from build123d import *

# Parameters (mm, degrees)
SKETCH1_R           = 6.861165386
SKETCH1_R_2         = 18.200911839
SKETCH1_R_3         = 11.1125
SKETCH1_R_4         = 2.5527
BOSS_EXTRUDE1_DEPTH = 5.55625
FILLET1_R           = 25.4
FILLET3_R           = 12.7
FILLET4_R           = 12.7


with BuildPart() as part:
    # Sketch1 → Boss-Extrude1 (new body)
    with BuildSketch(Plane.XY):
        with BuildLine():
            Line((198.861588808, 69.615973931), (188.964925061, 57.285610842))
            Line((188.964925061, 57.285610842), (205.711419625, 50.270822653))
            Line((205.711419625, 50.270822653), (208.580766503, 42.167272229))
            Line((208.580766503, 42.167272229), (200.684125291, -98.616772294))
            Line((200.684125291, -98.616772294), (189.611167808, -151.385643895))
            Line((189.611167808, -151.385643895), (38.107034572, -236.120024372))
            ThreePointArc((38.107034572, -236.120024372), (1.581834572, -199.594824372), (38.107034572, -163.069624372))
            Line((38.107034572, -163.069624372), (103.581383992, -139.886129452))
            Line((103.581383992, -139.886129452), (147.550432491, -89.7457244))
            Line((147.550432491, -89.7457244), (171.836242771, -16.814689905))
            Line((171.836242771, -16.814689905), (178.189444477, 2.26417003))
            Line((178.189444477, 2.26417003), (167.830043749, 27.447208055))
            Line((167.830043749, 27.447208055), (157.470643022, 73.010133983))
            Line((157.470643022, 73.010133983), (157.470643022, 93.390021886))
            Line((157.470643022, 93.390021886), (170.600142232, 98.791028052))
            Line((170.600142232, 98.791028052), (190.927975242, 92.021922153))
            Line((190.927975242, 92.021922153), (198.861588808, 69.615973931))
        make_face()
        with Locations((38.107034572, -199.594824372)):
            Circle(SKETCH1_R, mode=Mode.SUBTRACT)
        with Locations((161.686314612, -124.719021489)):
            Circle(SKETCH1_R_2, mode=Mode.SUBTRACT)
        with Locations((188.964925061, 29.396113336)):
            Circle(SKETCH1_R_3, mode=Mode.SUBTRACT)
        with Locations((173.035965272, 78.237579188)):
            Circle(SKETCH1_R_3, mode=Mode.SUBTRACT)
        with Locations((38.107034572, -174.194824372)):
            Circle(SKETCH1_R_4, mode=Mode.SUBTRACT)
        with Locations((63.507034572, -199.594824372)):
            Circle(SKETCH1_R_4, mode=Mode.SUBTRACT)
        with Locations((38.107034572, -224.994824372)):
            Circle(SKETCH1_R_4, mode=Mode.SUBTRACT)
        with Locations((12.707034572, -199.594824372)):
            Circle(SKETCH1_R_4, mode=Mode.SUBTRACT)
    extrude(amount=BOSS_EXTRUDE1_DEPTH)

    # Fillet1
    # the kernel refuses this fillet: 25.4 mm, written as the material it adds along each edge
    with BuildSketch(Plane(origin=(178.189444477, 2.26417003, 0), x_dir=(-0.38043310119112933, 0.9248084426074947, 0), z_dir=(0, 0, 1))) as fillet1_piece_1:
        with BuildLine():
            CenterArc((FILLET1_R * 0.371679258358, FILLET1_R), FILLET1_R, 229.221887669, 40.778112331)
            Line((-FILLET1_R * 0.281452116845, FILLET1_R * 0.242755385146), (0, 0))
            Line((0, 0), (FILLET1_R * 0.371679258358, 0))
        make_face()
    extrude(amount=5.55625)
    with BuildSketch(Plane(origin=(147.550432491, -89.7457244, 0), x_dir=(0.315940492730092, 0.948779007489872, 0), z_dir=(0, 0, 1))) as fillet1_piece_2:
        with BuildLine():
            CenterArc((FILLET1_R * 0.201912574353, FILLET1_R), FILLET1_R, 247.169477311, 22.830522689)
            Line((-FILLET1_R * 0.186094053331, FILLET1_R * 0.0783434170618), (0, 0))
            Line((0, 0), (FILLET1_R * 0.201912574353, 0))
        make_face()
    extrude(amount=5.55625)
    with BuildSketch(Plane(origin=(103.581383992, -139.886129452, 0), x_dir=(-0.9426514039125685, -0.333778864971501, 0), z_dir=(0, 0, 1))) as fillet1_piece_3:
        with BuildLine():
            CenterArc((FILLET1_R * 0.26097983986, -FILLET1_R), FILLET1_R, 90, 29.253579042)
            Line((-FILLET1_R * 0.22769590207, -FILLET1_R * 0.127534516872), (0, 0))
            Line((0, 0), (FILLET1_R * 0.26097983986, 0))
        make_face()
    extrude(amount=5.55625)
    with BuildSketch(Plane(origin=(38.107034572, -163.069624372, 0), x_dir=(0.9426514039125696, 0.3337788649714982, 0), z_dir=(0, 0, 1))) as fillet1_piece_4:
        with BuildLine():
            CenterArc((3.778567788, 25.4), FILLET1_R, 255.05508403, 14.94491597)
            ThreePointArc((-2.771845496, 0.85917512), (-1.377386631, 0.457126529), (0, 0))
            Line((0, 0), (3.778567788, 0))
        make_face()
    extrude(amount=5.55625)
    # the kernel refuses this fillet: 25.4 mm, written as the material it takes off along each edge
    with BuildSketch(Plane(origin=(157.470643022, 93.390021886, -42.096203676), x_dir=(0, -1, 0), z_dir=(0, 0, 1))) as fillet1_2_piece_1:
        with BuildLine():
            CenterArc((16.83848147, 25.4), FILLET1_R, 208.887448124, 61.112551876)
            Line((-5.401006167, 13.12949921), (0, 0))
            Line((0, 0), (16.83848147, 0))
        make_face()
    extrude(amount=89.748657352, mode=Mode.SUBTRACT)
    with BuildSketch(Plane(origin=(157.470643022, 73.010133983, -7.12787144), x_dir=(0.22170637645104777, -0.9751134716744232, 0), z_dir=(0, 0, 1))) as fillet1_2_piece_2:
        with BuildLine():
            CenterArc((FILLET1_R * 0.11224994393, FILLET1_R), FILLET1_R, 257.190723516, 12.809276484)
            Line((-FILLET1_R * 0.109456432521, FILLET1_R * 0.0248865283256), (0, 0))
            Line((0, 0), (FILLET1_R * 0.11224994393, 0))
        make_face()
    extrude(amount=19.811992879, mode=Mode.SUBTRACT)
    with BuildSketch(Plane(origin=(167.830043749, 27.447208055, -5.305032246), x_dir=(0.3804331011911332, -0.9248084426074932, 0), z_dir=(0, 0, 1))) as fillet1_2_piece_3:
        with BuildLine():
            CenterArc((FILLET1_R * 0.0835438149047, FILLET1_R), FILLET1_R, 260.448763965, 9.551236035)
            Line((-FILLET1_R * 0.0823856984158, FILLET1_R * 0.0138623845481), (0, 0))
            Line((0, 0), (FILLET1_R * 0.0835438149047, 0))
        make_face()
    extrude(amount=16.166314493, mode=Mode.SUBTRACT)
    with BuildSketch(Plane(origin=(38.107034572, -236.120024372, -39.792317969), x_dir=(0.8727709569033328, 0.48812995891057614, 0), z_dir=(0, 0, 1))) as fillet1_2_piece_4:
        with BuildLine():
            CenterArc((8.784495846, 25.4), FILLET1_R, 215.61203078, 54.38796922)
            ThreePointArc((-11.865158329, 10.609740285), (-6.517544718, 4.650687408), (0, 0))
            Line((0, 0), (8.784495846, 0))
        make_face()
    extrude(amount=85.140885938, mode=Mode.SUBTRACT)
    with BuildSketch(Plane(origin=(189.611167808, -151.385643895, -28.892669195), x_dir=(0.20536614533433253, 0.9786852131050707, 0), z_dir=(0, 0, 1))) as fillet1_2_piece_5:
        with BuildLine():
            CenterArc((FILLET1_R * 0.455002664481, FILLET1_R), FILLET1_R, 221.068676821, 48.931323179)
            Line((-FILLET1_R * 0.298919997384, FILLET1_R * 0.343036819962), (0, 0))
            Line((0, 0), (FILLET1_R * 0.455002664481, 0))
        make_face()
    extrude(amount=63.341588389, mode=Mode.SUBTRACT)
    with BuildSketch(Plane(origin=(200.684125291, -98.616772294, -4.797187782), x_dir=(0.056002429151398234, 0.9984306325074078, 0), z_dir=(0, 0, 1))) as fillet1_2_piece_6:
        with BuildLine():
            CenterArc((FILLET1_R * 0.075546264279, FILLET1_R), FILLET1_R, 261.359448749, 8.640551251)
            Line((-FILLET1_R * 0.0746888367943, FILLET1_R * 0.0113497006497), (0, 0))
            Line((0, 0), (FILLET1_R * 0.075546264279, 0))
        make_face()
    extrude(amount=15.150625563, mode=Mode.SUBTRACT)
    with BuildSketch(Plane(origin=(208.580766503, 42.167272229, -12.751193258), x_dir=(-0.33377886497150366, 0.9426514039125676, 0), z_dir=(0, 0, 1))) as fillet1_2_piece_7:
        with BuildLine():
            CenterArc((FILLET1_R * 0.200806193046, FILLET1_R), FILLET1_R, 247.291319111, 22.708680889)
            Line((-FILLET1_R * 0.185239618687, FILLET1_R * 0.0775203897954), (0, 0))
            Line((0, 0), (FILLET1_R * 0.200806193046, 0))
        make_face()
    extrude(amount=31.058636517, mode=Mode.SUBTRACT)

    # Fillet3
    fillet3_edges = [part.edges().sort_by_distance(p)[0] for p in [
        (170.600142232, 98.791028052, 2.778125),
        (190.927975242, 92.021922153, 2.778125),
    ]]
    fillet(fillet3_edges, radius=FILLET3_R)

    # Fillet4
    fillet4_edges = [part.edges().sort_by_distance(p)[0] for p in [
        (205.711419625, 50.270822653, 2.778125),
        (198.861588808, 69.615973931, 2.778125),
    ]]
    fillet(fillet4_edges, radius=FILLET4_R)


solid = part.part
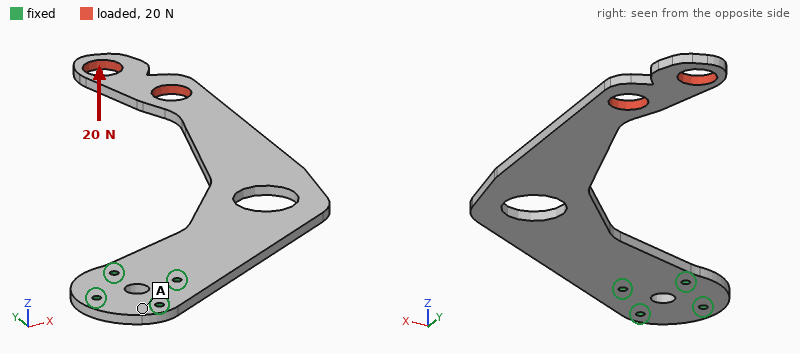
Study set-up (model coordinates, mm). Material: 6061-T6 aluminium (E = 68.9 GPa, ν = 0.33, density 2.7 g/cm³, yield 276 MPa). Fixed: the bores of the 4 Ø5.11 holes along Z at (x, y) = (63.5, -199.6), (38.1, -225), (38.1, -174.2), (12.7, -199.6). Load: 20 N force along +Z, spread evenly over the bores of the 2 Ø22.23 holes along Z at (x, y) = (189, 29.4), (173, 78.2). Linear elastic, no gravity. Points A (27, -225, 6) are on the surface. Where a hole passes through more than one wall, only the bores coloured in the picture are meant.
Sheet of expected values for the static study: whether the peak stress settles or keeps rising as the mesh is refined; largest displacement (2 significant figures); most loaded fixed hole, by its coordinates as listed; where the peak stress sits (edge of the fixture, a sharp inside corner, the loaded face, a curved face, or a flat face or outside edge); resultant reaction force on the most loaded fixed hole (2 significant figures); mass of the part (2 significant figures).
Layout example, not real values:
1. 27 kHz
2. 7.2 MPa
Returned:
1. keeps rising
2. 3.9 mm
3. (38.1, -174.2)
4. edge of the fixture
5. 48 N
6. 270 g
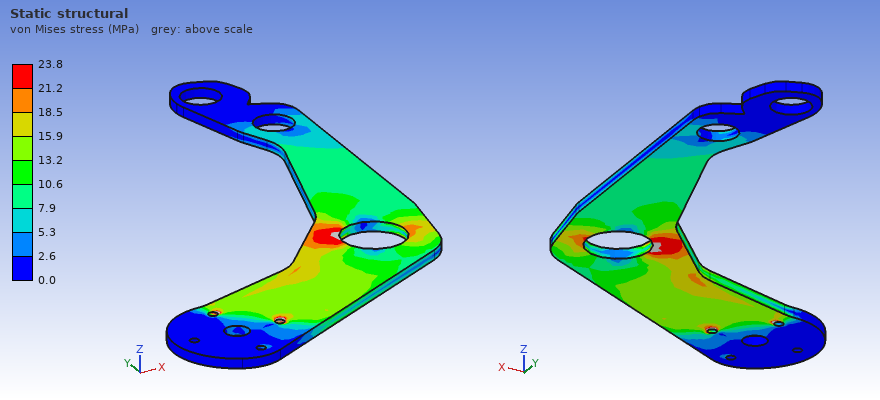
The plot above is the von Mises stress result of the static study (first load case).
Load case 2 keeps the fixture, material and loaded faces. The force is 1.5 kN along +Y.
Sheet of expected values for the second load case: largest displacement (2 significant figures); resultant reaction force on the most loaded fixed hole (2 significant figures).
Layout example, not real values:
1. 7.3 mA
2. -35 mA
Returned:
1. 0.71 mm
2. 3.7 kN
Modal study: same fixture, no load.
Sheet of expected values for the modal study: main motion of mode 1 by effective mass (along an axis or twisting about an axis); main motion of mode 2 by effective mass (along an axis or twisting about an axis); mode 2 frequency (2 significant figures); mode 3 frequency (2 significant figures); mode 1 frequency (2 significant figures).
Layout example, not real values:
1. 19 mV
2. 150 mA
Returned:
1. along Z
2. along Z
3. 200 Hz
4. 490 Hz
5. 54 Hz
